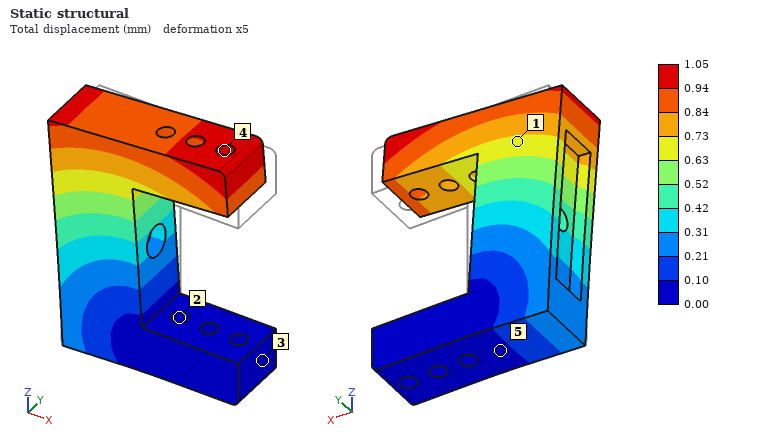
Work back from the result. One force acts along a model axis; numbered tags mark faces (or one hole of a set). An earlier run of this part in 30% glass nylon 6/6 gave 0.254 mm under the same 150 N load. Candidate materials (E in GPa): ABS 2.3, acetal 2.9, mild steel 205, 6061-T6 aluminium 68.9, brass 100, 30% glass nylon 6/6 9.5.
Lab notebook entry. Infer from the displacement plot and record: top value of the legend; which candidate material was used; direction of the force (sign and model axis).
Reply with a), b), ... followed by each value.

a) 1.05 mm
b) ABS
c) -X
